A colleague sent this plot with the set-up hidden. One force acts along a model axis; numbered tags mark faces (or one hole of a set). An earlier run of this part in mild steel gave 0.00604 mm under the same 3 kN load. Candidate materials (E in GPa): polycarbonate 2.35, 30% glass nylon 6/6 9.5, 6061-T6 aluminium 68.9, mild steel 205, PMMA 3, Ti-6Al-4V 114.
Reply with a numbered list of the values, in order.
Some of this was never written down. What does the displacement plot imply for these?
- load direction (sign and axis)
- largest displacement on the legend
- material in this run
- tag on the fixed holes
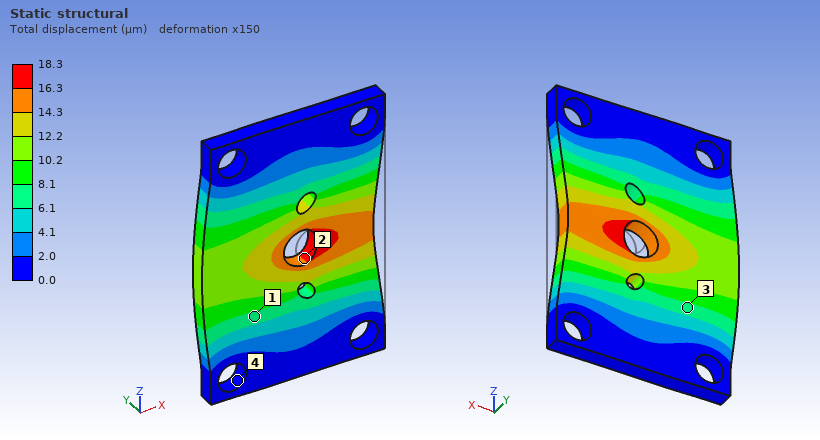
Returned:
1. -X
2. 18.3 µm
3. 6061-T6 aluminium
4. 4
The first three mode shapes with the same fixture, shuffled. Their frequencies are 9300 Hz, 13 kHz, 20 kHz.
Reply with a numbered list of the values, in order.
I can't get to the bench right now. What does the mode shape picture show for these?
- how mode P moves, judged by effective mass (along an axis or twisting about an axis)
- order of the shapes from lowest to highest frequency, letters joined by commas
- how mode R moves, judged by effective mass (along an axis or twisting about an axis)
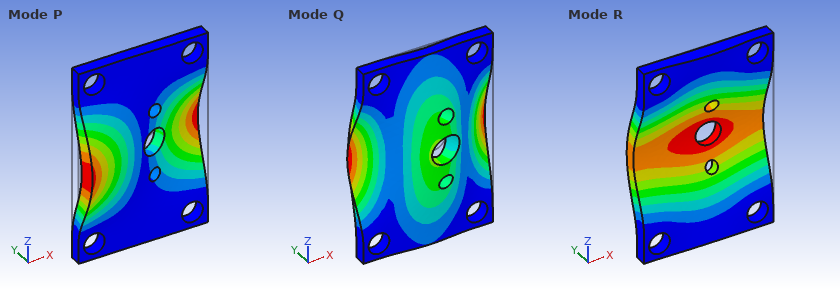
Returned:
1. twisting about Z
2. R, P, Q
3. along Y
